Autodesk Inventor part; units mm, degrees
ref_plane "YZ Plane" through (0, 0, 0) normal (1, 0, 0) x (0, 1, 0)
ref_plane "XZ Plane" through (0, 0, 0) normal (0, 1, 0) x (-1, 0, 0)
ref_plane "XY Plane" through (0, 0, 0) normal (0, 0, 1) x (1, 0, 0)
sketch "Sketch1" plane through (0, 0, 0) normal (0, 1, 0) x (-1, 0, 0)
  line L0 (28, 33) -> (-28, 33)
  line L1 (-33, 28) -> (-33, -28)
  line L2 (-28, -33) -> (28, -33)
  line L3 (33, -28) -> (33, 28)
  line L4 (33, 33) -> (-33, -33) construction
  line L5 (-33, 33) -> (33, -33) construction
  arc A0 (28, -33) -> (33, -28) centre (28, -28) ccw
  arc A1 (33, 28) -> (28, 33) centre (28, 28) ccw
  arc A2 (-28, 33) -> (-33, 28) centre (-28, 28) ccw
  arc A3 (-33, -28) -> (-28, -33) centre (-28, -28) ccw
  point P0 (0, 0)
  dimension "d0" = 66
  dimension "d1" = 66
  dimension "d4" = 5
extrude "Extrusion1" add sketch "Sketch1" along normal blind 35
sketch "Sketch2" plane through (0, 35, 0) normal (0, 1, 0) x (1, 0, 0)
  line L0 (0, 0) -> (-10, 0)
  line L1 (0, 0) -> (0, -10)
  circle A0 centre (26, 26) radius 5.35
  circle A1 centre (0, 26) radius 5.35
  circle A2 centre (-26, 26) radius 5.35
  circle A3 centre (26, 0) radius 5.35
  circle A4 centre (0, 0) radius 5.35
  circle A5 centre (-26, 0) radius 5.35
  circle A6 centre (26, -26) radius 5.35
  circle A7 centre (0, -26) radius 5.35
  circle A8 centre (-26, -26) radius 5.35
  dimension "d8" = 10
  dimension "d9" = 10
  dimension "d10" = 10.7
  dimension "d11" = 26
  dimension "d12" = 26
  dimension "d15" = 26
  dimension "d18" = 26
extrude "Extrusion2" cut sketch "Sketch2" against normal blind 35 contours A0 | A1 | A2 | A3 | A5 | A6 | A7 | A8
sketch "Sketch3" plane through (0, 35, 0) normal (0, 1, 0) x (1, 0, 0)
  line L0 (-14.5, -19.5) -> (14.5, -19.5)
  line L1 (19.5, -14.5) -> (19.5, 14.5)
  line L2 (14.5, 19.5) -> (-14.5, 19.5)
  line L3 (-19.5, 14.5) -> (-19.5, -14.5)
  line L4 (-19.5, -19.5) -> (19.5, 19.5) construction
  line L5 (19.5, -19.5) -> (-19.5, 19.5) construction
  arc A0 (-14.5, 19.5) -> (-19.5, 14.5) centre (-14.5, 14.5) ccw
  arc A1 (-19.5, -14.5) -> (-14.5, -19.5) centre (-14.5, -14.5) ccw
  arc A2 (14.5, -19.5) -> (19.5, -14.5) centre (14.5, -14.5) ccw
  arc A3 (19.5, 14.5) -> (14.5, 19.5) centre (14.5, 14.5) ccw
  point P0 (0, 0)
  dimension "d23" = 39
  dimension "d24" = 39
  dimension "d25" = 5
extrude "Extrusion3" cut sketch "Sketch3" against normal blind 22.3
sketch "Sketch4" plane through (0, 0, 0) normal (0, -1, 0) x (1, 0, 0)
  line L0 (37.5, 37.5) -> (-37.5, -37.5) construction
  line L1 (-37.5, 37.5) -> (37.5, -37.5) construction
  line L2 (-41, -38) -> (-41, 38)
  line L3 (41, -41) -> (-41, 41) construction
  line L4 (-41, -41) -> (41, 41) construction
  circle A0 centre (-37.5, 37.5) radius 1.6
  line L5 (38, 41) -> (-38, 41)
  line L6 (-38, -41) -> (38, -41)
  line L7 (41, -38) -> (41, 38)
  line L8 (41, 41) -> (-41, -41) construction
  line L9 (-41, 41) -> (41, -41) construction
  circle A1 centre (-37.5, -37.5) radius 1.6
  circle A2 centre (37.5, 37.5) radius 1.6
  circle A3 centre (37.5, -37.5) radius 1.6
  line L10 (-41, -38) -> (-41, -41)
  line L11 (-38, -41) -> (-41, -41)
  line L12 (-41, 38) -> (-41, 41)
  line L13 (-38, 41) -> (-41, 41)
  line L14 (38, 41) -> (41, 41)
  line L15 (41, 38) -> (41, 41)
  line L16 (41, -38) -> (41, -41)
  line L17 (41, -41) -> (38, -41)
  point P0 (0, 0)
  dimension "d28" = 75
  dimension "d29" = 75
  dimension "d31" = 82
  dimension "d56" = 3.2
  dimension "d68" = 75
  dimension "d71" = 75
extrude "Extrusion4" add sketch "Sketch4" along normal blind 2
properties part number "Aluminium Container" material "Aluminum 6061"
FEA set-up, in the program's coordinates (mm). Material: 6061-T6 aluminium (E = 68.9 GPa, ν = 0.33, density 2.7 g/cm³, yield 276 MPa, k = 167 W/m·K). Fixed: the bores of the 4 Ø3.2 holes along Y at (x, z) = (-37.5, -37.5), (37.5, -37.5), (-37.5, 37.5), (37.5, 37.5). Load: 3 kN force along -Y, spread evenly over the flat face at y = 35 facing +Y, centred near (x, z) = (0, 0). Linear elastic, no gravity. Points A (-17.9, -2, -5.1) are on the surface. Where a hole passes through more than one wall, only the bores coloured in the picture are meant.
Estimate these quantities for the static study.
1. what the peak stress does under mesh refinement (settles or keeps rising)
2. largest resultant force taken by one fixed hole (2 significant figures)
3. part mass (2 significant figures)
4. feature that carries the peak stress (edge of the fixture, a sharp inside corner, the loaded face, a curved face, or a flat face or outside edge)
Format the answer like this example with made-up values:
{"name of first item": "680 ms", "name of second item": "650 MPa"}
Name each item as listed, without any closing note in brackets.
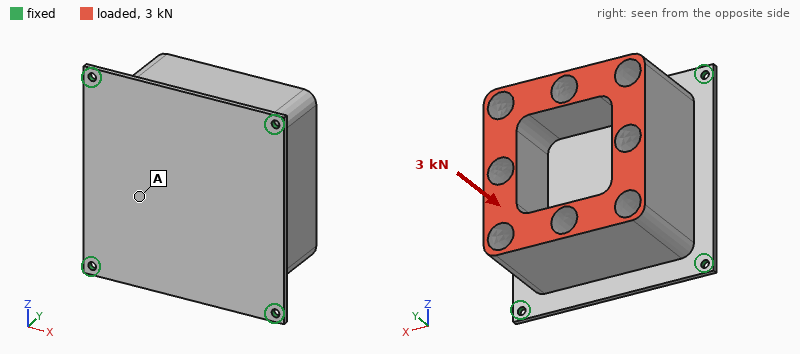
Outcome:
{"what the peak stress does under mesh refinement": "keeps rising", "largest resultant force taken by one fixed hole": "830 N", "part mass": "290 g", "feature that carries the peak stress": "edge of the fixture"}
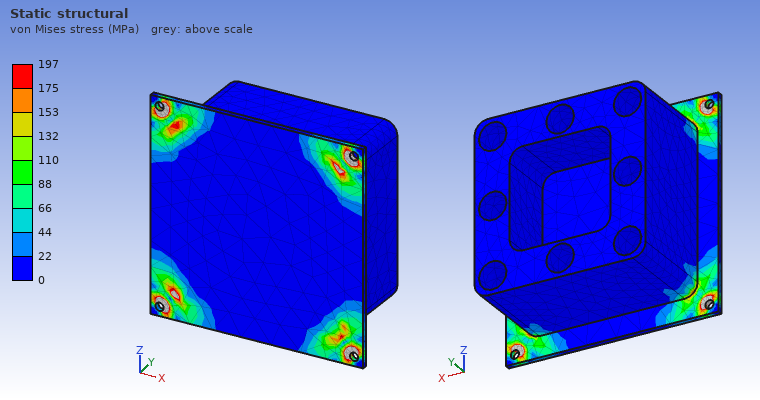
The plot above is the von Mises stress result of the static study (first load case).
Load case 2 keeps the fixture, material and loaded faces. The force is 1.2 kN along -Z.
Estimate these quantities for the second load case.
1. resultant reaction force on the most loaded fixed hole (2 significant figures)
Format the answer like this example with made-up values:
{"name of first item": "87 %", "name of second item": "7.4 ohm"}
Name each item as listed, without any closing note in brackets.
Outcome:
{"resultant reaction force on the most loaded fixed hole": "470 N"}
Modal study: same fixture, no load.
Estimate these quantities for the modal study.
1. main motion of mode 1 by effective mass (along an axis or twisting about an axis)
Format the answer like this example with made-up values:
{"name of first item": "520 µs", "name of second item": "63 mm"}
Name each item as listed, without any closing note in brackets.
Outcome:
{"main motion of mode 1 by effective mass": "along Y"}
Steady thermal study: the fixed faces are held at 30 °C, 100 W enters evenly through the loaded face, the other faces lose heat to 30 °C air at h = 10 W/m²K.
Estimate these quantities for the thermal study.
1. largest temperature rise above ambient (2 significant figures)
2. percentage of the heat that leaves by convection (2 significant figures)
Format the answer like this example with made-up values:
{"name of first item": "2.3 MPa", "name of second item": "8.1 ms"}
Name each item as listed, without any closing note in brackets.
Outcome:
{"largest temperature rise above ambient": "62 K", "percentage of the heat that leaves by convection": "18 %"}
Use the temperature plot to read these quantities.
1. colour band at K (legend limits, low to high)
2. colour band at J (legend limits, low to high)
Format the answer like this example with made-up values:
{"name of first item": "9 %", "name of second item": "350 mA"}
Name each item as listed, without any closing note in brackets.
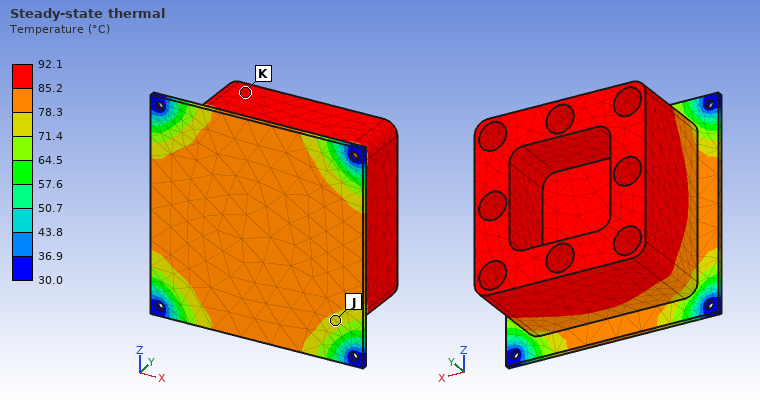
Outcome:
{"colour band at K": "85.2 to 92.1 °C", "colour band at J": "71.4 to 78.3 °C"}
